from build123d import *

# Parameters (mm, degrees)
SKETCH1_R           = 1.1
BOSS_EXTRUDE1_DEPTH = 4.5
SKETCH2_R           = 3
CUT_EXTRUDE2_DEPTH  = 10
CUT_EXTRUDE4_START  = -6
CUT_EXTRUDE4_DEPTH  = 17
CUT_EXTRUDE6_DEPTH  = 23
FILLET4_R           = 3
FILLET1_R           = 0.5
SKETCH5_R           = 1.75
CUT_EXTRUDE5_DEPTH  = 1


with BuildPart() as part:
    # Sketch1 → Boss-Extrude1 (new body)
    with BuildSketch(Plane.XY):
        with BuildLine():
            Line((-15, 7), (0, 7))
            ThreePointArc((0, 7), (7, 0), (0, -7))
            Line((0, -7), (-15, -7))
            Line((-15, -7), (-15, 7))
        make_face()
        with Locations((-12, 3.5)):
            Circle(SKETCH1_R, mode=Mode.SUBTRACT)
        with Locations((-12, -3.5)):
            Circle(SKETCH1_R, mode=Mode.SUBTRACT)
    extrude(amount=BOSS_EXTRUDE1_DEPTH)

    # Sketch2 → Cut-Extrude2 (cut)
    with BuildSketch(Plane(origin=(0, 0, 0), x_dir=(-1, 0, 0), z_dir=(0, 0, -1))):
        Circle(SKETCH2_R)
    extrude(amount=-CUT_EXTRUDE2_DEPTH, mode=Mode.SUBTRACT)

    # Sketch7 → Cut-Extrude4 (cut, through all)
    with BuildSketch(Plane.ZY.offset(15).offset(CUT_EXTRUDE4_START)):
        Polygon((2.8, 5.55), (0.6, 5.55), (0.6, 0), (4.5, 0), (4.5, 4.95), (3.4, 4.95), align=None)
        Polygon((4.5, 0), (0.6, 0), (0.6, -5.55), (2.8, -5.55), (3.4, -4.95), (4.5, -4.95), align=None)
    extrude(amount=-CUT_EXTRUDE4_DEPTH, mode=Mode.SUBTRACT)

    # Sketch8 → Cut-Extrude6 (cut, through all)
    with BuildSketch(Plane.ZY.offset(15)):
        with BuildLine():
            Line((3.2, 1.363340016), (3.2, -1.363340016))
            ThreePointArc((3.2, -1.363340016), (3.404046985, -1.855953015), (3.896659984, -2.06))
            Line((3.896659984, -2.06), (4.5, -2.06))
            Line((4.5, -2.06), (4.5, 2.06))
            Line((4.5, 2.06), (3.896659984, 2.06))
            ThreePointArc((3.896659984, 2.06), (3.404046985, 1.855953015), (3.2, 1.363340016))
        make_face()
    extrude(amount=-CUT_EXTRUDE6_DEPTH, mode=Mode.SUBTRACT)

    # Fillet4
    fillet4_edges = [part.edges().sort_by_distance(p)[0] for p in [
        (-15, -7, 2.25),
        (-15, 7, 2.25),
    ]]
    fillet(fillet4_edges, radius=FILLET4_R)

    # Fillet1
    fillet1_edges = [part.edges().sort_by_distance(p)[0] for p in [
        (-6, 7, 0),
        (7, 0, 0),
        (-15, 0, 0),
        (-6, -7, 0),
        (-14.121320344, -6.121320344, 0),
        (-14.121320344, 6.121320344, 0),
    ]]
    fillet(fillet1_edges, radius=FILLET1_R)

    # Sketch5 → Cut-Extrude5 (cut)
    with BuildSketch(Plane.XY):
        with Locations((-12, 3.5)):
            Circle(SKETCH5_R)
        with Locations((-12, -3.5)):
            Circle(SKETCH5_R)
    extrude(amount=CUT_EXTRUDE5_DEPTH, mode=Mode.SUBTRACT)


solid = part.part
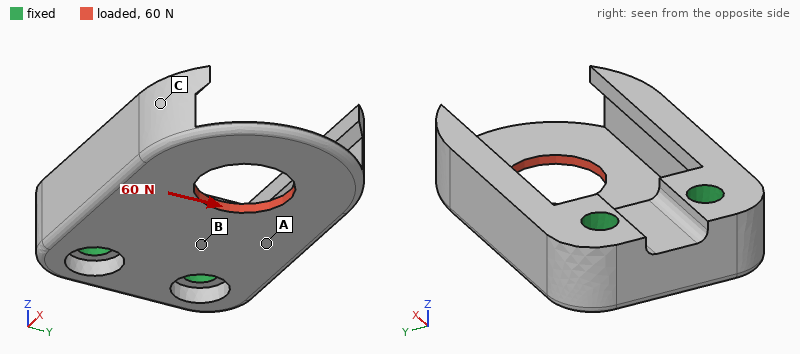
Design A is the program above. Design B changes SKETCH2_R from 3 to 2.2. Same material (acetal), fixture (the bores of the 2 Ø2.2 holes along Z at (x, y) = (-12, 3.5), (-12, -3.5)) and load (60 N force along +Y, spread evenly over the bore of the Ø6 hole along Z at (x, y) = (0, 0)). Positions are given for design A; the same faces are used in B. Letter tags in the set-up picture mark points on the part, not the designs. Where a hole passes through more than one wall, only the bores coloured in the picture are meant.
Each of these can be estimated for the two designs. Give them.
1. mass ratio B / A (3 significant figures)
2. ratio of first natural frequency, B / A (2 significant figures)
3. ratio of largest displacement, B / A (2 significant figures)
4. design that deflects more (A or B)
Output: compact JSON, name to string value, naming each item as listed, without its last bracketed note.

{"mass ratio B / A": "1.01", "ratio of first natural frequency, B / A": "0.98", "ratio of largest displacement, B / A": "0.88", "design that deflects more": "A"}
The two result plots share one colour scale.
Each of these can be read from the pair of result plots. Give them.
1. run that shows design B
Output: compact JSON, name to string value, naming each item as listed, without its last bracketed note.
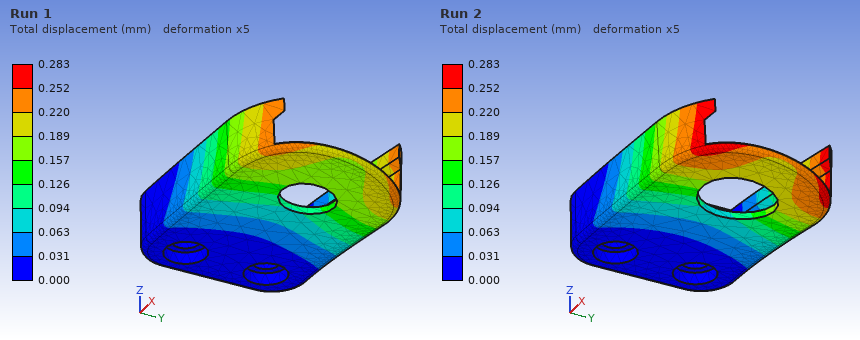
{"run that shows design B": "Run 1"}
